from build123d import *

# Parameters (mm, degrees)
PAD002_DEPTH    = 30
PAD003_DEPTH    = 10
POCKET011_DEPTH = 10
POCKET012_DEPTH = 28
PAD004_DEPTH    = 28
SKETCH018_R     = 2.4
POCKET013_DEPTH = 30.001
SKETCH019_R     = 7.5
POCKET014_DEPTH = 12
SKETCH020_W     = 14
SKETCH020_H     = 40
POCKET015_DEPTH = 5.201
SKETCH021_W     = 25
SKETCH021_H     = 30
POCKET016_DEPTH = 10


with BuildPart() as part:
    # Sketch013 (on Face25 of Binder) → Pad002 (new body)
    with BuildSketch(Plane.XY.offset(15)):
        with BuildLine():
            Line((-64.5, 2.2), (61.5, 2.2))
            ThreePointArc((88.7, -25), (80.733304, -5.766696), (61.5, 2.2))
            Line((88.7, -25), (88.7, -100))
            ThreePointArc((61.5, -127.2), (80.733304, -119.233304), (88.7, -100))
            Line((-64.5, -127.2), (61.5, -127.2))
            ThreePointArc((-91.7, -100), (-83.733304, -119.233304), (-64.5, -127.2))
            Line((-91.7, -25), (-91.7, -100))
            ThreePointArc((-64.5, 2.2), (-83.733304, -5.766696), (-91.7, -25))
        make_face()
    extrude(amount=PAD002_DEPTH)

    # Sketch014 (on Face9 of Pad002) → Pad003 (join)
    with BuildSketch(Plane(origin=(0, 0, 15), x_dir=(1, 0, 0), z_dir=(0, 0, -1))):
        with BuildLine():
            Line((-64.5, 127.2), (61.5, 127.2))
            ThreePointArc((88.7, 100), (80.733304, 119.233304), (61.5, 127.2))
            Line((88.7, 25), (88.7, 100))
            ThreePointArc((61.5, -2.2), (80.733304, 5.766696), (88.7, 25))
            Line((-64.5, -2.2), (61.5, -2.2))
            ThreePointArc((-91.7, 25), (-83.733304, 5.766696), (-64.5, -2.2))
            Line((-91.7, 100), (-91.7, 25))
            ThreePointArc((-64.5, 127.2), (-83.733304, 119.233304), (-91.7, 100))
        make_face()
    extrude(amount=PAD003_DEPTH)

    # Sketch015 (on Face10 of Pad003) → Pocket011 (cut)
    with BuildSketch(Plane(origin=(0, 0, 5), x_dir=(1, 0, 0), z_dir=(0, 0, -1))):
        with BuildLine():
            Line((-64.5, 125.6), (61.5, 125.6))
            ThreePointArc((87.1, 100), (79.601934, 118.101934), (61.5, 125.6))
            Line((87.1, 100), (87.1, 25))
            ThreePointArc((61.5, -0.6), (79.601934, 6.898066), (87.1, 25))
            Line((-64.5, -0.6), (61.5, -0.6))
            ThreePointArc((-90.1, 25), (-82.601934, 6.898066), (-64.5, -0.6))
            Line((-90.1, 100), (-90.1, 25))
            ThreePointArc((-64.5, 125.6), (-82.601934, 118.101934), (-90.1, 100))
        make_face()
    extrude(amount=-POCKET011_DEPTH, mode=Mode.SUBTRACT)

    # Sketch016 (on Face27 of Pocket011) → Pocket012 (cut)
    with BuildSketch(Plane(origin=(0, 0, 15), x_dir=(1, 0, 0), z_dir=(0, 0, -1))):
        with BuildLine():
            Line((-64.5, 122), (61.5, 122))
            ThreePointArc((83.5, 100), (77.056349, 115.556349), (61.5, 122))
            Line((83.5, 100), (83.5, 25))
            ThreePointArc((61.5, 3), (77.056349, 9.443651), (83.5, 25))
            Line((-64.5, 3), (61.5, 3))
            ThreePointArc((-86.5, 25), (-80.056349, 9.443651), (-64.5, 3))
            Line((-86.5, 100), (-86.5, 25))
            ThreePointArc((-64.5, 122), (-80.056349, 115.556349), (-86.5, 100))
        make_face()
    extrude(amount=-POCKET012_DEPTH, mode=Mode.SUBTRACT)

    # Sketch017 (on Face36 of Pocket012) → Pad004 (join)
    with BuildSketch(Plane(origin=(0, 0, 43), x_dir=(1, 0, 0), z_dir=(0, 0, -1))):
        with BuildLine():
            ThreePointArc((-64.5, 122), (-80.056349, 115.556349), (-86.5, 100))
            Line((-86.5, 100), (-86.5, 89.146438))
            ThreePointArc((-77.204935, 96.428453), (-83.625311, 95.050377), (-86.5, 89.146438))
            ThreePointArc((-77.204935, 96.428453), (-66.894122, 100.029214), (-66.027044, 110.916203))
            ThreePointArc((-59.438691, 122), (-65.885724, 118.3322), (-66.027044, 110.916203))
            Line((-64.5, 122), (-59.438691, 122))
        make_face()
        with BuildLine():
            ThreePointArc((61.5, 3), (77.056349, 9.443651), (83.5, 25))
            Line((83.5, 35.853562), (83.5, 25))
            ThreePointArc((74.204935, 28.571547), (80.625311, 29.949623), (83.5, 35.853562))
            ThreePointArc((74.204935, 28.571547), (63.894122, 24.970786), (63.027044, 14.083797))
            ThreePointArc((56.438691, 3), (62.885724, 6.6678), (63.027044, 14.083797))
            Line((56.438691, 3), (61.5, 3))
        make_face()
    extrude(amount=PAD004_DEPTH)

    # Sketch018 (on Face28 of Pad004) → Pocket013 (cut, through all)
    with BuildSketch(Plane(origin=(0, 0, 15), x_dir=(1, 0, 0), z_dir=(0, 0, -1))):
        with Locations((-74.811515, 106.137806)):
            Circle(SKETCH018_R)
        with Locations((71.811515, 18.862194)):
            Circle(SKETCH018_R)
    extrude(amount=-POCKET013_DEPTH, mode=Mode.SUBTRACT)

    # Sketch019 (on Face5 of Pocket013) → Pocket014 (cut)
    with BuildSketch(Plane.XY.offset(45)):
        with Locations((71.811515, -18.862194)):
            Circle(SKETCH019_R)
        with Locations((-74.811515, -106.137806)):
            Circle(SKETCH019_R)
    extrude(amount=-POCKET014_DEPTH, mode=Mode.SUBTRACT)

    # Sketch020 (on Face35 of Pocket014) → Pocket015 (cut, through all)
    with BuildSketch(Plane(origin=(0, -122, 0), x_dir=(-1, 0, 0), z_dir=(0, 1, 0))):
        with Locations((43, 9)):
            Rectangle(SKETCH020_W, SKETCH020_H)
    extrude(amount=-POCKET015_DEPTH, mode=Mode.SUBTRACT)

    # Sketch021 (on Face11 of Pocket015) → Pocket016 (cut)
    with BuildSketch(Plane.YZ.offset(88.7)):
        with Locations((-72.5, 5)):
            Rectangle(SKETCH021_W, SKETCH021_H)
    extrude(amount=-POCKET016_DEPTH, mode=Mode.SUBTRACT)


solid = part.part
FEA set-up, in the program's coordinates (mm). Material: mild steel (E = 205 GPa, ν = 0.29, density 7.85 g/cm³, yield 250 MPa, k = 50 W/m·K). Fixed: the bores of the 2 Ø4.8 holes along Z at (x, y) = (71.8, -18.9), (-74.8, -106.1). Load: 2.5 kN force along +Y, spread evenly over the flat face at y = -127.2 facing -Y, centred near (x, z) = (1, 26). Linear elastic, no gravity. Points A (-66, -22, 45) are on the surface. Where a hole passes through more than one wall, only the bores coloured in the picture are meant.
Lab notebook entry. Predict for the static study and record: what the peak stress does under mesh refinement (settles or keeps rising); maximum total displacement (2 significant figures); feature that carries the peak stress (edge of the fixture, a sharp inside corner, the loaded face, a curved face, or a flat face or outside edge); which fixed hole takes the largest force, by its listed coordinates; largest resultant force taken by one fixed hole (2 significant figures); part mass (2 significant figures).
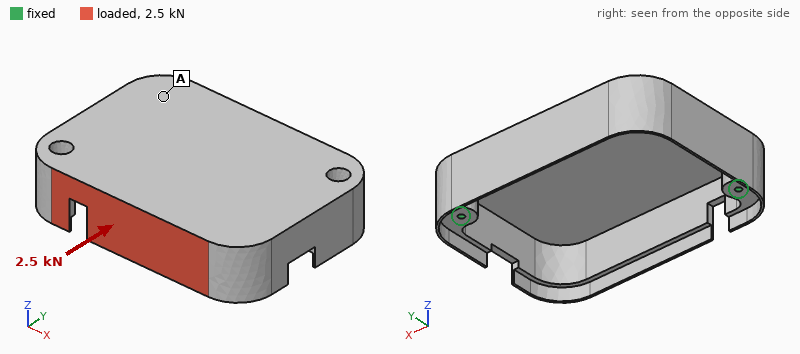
keeps rising
0.33 mm
a sharp inside corner
(71.8, -18.9)
1.4 kN
1.2 kg
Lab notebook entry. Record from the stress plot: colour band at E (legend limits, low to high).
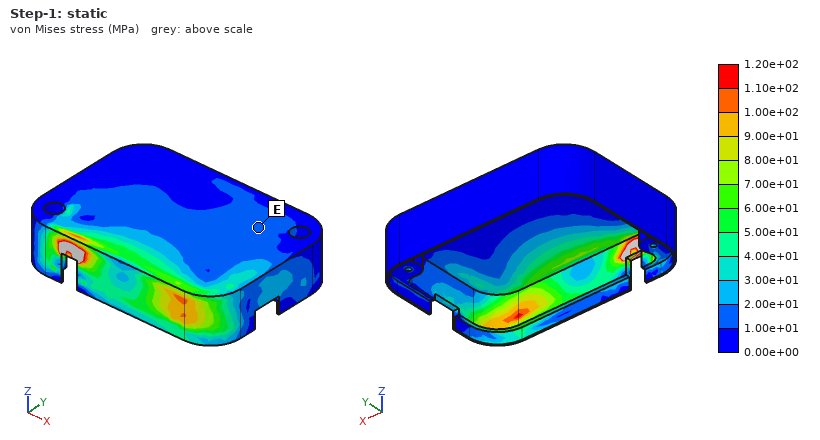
1.00e+01 to 2.00e+01 MPa
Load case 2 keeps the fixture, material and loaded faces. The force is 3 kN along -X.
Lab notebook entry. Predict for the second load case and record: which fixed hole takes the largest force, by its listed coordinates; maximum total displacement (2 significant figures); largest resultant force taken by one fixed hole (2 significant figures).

(-74.8, -106.1)
50 µm
2.8 kN
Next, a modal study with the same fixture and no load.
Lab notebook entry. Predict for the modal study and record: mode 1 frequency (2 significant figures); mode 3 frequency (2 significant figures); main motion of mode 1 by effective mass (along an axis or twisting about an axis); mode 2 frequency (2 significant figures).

890 Hz
1600 Hz
along Z
1200 Hz
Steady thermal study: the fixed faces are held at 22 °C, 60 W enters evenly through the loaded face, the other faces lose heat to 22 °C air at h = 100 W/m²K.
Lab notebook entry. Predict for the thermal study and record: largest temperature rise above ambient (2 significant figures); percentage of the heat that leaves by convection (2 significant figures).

57 K
87 %
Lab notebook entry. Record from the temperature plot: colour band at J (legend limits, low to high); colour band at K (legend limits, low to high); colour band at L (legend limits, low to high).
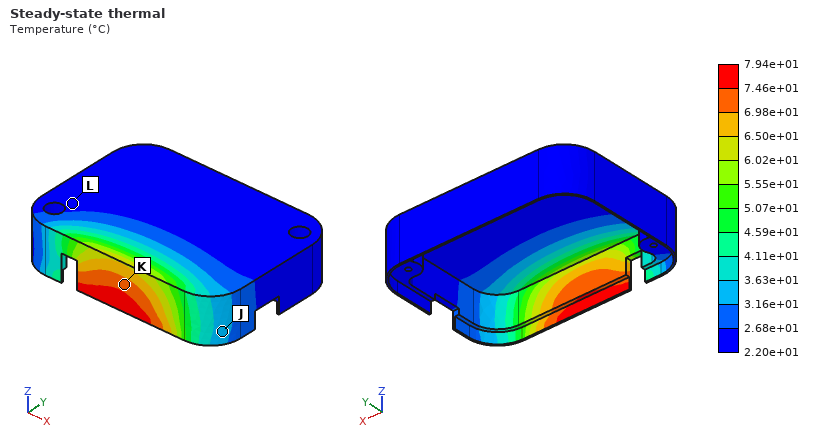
3.16e+01 to 3.63e+01 °C
6.98e+01 to 7.46e+01 °C
2.20e+01 to 2.68e+01 °C
